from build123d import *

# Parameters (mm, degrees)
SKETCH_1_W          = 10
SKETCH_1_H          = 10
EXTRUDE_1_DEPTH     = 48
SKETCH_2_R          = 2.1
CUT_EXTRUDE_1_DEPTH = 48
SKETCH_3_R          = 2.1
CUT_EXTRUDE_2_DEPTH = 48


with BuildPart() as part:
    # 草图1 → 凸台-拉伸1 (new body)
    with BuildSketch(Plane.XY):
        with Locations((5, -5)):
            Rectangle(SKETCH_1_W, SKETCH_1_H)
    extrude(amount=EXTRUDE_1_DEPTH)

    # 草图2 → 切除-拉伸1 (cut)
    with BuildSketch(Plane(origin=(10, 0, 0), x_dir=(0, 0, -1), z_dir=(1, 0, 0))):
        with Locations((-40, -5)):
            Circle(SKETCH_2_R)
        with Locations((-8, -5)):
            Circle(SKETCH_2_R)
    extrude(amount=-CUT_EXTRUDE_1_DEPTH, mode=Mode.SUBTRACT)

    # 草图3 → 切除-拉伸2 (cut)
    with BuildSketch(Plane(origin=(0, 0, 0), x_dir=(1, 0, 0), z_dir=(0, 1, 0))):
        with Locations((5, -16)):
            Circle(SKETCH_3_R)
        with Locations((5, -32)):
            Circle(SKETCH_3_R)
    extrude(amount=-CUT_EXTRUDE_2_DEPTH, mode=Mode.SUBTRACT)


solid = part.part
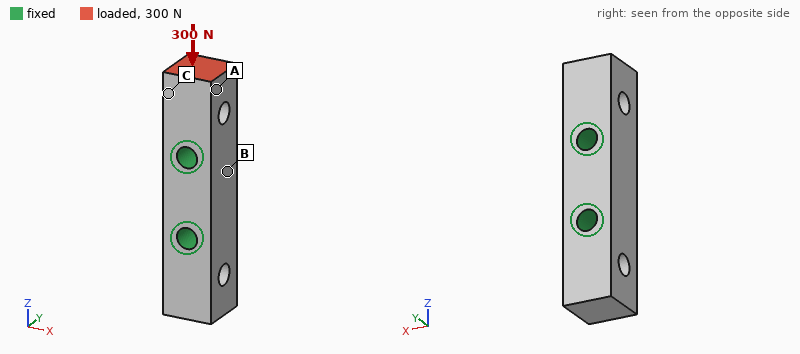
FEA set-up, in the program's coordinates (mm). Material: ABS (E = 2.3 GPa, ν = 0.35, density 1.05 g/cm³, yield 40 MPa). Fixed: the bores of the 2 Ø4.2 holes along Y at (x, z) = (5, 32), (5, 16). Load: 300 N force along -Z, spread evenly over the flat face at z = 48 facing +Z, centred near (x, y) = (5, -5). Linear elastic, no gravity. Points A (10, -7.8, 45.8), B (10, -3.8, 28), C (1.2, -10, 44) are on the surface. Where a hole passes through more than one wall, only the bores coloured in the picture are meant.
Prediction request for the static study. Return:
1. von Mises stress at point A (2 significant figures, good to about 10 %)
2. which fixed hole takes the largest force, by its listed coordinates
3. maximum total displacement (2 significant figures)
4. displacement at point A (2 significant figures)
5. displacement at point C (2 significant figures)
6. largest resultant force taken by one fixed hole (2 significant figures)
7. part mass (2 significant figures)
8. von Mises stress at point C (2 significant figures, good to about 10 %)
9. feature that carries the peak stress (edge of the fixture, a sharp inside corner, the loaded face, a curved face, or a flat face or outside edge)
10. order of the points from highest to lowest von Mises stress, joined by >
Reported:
3.3 MPa
(5, 32)
28 µm
24 µm
20 µm
290 N
4.5 g
4.2 MPa
a curved face
C > A > B
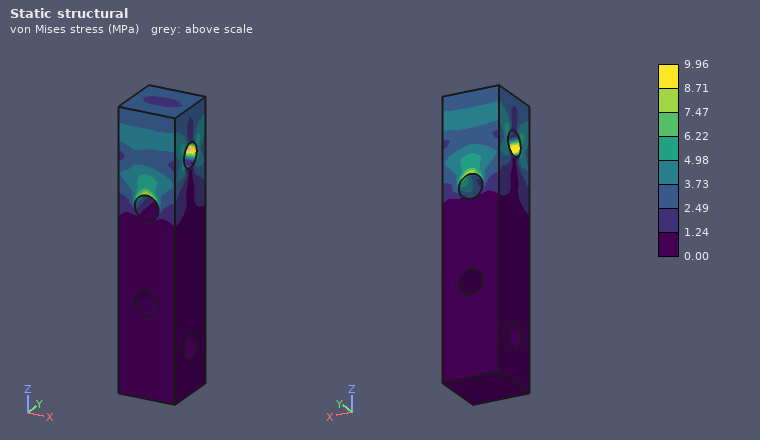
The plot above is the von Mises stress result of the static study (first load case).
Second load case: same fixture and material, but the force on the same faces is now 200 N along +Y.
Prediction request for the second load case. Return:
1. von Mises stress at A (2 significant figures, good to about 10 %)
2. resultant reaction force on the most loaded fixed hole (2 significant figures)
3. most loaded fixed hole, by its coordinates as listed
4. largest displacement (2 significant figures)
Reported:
3.9 MPa
210 N
(5, 32)
0.21 mm
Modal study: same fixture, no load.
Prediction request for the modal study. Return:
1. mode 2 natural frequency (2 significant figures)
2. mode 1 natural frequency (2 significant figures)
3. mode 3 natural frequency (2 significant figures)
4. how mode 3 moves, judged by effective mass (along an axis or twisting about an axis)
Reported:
6500 Hz
6500 Hz
7400 Hz
along Y
